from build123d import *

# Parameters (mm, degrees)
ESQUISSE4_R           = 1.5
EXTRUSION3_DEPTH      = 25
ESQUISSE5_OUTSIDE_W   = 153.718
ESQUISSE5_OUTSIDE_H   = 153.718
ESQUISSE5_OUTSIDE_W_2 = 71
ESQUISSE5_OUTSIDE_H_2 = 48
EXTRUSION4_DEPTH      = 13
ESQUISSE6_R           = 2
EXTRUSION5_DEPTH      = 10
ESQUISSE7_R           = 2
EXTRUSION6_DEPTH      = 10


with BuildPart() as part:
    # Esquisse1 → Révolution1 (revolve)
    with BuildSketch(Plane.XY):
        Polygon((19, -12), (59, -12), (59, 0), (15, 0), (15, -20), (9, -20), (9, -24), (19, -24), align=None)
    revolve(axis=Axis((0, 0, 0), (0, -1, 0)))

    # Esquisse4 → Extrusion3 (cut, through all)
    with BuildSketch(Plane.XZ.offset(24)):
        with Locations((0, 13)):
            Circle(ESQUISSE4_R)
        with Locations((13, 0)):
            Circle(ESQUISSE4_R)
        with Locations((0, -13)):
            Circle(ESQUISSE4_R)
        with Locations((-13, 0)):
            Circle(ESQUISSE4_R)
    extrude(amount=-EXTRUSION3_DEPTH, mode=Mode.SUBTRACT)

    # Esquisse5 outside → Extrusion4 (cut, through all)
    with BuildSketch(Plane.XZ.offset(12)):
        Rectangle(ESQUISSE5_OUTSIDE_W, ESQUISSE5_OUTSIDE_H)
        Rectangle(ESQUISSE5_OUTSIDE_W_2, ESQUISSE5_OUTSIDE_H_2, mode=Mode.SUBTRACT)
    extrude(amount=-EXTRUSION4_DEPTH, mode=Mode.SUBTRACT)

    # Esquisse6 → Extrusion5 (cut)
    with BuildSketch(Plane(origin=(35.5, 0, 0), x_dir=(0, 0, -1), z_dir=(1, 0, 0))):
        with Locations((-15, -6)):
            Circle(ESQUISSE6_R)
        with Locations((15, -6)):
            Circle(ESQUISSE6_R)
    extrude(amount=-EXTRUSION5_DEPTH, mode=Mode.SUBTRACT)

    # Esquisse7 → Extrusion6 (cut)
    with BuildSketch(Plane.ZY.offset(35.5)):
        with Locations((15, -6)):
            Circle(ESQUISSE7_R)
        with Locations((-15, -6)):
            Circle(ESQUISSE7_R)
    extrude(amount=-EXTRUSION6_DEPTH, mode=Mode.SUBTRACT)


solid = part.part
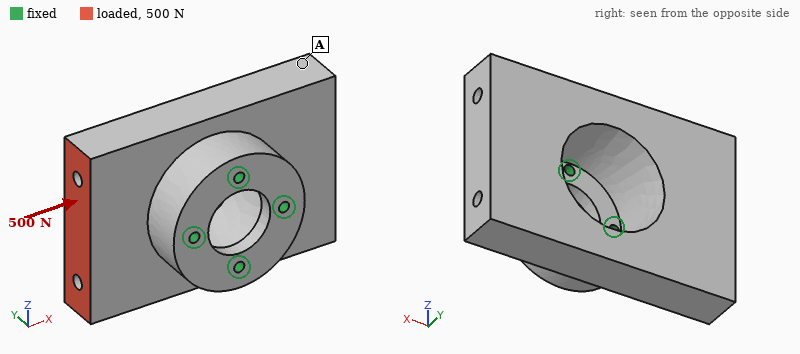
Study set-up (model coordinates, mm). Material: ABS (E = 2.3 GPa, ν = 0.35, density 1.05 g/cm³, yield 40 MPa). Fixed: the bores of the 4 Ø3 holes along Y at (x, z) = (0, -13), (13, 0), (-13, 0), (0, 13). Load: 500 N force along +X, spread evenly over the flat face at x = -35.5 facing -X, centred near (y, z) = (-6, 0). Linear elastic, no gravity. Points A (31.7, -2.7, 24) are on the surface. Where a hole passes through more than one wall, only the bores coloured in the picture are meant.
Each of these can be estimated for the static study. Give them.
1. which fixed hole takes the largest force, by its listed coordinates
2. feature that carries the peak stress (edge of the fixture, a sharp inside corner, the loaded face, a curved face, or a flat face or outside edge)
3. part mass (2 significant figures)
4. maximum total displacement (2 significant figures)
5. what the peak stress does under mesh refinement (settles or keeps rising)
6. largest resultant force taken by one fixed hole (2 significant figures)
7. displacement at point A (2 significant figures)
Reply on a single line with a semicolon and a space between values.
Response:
(-13, 0); edge of the fixture; 41 g; 0.21 mm; keeps rising; 260 N; 0.16 mm
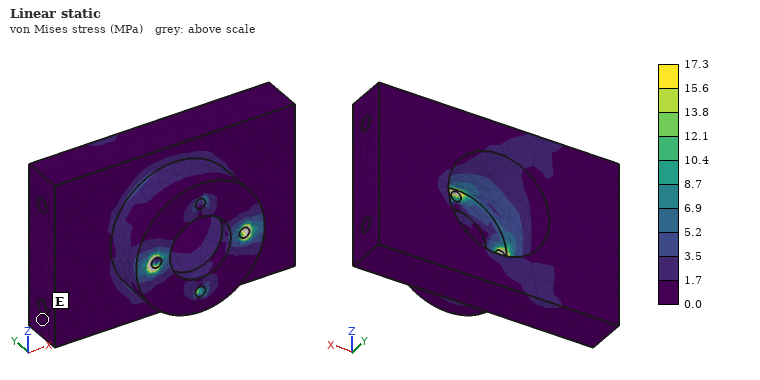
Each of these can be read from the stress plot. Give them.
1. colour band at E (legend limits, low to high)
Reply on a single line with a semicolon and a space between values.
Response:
0.0 to 1.7 MPa
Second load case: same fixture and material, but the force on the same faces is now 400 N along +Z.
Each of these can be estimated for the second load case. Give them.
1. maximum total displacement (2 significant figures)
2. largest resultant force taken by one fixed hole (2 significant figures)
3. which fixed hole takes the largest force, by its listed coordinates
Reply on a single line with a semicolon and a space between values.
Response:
0.25 mm; 420 N; (-13, 0)
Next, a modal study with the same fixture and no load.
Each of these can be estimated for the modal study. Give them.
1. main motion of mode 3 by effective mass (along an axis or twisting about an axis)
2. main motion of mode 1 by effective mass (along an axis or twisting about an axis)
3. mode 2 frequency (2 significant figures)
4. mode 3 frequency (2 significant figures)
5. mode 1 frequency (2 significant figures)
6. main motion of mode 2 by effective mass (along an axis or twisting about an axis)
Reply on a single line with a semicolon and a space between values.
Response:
twisting about Y; along X; 1600 Hz; 2300 Hz; 1400 Hz; along Z
